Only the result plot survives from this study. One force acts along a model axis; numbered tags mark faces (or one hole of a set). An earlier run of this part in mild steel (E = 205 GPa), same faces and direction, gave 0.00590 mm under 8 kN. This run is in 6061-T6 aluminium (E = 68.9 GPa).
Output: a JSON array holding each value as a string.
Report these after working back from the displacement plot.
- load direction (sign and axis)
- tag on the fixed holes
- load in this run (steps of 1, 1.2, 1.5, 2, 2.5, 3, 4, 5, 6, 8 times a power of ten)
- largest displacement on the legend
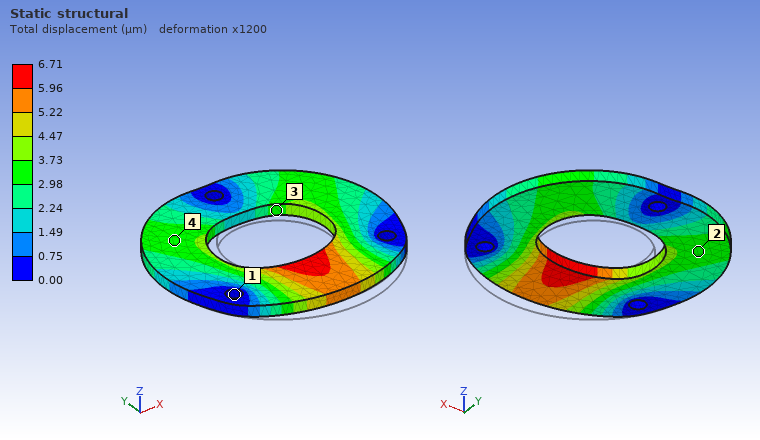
["+Y", "1", "3 kN", "6.71 µm"]
